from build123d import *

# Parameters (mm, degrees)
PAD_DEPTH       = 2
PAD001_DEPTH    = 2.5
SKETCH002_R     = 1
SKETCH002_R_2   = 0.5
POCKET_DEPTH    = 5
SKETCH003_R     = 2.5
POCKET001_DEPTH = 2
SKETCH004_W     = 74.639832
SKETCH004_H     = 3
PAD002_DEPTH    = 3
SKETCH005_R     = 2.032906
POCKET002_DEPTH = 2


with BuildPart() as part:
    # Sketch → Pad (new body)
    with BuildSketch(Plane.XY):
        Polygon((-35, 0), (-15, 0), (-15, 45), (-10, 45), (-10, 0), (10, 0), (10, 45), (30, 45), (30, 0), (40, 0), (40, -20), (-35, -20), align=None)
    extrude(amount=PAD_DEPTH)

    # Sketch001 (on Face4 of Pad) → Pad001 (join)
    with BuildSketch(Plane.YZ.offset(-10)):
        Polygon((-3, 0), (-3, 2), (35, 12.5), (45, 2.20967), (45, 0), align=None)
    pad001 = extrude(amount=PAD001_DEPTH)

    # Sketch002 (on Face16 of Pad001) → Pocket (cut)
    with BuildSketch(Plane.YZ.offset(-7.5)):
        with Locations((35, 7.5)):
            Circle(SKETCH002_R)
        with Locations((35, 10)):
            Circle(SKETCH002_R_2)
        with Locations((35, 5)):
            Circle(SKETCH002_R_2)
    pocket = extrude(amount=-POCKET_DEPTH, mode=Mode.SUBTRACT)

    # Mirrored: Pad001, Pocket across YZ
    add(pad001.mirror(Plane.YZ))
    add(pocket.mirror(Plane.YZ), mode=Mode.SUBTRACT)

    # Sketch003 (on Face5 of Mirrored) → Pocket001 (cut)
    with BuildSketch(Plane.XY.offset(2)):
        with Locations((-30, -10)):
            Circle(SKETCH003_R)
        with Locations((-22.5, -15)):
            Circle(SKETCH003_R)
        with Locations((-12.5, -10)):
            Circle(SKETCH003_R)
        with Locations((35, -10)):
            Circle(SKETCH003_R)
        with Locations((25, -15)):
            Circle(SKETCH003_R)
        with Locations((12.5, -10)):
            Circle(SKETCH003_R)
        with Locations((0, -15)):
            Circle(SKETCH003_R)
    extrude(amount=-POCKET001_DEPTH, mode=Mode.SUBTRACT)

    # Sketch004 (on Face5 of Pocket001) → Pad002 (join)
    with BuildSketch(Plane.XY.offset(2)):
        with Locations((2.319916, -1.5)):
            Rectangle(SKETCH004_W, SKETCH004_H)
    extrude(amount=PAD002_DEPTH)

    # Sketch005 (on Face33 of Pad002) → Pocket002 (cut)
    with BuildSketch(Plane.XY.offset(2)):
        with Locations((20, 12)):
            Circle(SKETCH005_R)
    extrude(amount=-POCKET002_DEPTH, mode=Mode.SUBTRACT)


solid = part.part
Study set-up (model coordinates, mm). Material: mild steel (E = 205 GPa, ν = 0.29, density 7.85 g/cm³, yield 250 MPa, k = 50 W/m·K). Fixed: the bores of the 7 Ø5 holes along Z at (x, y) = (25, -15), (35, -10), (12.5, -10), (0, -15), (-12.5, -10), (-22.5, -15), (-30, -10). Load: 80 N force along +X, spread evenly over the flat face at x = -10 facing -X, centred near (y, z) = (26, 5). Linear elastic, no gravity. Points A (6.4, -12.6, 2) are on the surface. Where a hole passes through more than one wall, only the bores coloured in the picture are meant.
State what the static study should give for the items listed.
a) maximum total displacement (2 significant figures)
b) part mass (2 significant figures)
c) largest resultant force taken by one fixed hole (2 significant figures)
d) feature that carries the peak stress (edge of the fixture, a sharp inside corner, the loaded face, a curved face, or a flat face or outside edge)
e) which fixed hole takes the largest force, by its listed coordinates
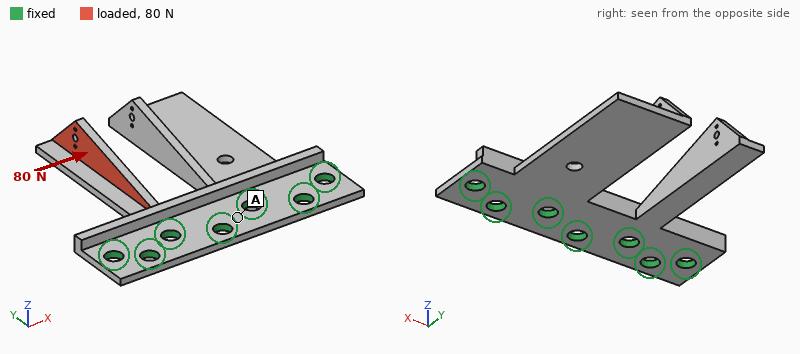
0.10 mm
57 g
93 N
a flat face or outside edge
(0, -15)
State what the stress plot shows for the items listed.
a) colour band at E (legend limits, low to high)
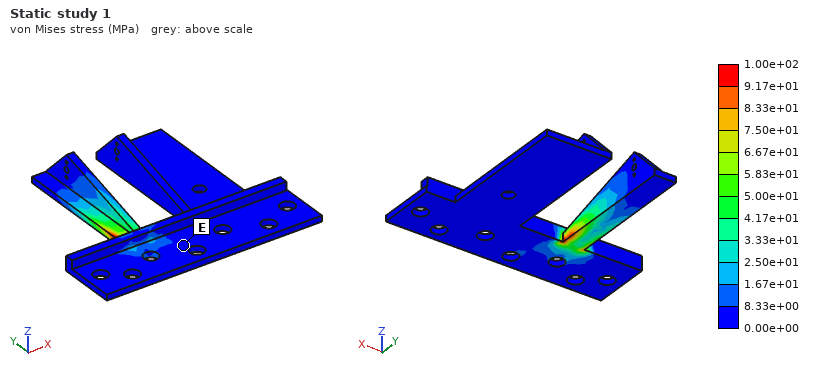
0.00e+00 to 8.33e+00 MPa
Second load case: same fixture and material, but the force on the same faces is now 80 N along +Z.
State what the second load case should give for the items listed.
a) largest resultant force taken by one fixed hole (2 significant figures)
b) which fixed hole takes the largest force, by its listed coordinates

92 N
(12.5, -10)
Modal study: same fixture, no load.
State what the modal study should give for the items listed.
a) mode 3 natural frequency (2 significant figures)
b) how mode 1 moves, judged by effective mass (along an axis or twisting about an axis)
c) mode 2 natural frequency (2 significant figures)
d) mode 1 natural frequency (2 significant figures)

2100 Hz
along Z
840 Hz
710 Hz
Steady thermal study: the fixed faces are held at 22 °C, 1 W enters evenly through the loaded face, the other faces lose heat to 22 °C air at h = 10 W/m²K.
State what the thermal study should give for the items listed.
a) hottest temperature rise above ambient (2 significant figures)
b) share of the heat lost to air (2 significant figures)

21 K
21 %
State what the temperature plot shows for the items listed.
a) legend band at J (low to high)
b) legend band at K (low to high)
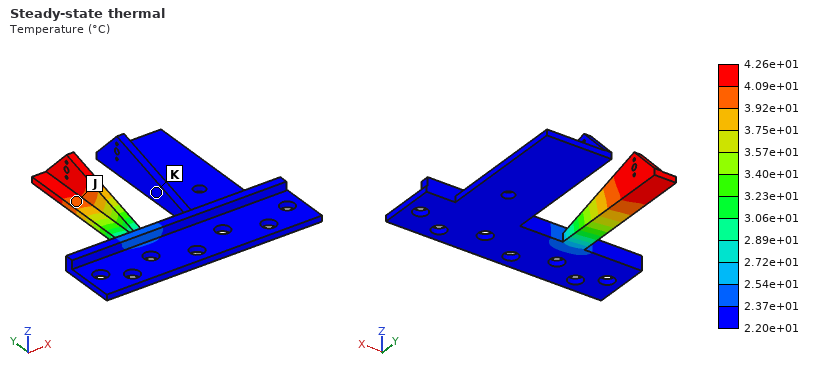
3.92e+01 to 4.09e+01 °C
2.20e+01 to 2.37e+01 °C
